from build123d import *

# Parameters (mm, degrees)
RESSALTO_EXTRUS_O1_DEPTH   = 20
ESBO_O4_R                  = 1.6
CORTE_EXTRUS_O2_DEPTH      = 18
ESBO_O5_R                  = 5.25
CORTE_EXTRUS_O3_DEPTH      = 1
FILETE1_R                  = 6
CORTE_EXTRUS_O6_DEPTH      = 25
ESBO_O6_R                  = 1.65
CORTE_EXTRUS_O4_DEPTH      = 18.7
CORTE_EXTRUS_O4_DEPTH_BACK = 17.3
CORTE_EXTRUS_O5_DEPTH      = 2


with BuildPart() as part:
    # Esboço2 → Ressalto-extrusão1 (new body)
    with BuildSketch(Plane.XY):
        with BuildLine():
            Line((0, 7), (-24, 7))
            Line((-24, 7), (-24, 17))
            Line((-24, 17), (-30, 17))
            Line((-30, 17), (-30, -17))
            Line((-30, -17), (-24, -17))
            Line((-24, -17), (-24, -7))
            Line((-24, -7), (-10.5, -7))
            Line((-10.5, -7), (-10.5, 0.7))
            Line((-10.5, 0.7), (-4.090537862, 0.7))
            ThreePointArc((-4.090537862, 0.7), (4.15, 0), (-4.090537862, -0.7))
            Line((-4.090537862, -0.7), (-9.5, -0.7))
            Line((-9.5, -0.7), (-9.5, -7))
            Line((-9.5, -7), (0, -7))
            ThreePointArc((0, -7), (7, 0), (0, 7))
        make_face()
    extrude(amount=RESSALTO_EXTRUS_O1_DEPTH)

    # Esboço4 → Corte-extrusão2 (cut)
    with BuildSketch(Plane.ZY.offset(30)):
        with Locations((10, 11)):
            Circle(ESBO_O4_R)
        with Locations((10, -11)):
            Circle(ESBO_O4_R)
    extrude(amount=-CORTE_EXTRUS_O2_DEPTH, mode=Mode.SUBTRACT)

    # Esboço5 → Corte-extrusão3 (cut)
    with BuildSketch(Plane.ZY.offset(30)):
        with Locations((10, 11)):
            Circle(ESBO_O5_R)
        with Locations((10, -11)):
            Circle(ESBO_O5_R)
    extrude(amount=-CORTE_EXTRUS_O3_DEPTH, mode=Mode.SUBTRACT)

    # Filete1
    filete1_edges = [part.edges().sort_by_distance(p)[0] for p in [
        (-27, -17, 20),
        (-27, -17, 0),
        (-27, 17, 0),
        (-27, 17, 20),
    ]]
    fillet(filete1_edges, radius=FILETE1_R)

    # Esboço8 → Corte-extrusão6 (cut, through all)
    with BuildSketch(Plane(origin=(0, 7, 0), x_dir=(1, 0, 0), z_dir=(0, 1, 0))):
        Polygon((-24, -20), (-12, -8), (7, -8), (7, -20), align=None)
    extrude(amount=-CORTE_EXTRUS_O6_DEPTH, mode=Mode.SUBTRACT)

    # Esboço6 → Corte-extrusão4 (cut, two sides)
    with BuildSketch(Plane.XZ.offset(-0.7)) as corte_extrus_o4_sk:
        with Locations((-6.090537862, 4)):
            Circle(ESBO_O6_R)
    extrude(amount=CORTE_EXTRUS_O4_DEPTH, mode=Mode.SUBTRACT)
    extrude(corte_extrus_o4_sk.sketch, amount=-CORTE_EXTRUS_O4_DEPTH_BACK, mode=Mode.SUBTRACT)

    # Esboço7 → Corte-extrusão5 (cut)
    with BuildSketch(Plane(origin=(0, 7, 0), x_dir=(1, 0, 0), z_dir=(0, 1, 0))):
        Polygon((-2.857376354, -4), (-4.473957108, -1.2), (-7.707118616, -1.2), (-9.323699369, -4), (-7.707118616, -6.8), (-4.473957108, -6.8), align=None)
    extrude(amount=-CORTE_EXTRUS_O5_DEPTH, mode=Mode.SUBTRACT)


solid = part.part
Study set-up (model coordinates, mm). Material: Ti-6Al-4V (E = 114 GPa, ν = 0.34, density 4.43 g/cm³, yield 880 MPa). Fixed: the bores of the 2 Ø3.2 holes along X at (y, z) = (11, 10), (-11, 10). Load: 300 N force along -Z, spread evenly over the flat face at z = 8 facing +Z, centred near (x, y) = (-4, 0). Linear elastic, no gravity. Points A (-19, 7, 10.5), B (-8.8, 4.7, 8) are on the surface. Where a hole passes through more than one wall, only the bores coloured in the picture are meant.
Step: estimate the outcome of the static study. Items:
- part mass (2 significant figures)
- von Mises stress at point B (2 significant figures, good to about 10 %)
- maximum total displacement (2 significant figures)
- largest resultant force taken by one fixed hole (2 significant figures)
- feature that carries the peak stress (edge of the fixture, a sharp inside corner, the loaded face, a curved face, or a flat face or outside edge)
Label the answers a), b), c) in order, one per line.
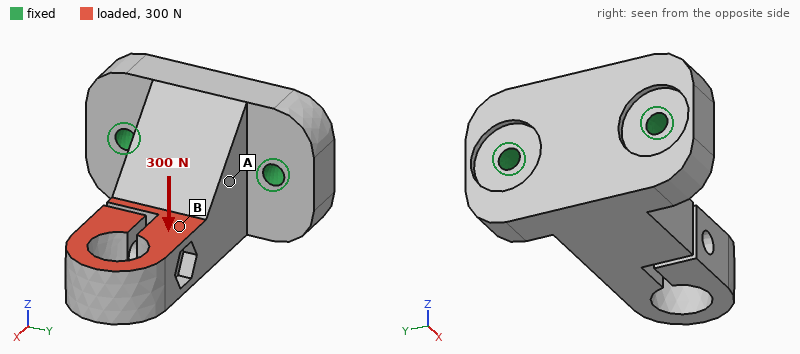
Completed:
a) 32 g
b) 39 MPa
c) 0.15 mm
d) 150 N
e) a curved face
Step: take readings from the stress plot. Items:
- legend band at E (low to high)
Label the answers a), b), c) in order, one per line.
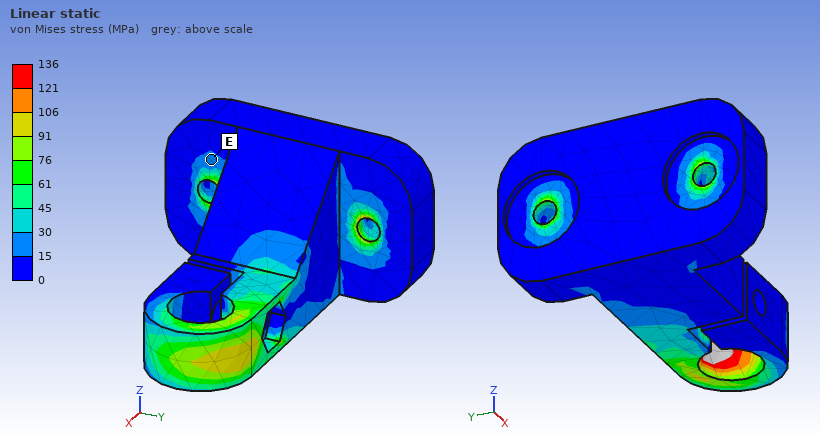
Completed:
a) 15 to 30 MPa
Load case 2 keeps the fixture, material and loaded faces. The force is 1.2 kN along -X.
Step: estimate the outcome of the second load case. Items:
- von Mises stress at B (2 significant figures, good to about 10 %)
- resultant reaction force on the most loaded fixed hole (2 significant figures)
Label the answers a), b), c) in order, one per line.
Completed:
a) 70 MPa
b) 620 N
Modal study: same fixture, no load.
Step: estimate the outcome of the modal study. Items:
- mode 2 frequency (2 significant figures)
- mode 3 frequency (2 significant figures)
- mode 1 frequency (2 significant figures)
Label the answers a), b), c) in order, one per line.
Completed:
a) 3500 Hz
b) 5400 Hz
c) 3300 Hz
